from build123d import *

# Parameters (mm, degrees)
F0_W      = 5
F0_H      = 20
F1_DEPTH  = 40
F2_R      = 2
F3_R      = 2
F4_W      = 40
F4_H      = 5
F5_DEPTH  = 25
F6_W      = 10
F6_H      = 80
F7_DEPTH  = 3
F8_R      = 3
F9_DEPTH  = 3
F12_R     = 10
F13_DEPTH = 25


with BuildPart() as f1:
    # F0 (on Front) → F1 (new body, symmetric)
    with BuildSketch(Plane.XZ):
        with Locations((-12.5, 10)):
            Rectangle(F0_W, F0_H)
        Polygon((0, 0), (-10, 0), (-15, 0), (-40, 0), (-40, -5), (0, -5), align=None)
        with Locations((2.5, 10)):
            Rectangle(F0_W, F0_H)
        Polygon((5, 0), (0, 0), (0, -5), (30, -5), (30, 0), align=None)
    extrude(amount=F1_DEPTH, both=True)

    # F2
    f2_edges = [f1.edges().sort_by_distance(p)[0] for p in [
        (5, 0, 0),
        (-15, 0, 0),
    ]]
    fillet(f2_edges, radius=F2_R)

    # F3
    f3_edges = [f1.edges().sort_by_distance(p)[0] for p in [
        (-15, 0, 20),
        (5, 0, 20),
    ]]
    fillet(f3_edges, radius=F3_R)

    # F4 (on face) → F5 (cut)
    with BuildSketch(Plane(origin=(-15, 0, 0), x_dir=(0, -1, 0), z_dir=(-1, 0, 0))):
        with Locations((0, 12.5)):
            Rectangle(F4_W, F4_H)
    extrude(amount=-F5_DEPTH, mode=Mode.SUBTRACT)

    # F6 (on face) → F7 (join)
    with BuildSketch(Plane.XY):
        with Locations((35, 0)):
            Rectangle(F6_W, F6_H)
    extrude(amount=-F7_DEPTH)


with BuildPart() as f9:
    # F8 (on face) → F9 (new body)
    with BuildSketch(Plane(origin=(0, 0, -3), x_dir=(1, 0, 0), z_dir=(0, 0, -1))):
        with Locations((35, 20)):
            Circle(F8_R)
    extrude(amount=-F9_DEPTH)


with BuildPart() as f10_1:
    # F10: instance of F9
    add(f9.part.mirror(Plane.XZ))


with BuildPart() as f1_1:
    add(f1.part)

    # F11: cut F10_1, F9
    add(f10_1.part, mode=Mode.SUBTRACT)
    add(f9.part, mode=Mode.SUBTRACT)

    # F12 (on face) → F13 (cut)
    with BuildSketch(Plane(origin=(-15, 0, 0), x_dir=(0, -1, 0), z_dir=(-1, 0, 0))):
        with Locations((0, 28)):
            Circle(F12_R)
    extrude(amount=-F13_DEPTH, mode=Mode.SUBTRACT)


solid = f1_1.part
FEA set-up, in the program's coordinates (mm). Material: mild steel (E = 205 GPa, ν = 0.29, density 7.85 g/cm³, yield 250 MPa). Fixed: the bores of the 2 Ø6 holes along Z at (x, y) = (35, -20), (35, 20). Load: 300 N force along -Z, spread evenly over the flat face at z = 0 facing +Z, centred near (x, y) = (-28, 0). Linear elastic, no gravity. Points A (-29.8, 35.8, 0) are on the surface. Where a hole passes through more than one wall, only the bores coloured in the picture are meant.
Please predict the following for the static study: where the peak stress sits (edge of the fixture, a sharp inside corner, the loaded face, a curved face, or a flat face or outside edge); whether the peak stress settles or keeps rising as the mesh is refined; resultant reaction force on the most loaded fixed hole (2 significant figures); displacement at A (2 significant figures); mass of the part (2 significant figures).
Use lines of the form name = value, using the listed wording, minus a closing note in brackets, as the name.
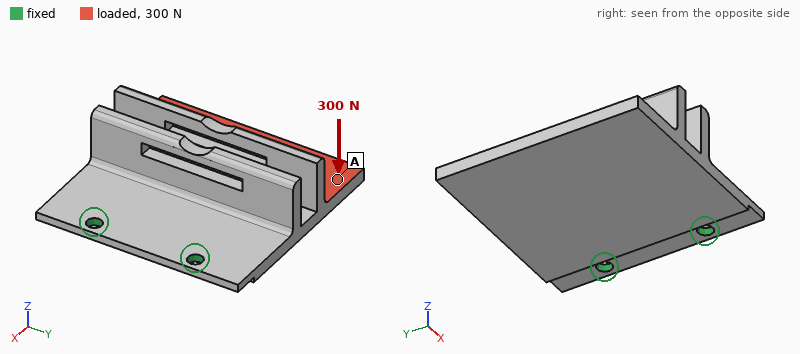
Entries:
where the peak stress sits = edge of the fixture
whether the peak stress settles or keeps rising as the mesh is refined = keeps rising
resultant reaction force on the most loaded fixed hole = 150 N
displacement at A = 0.32 mm
mass of the part = 350 g
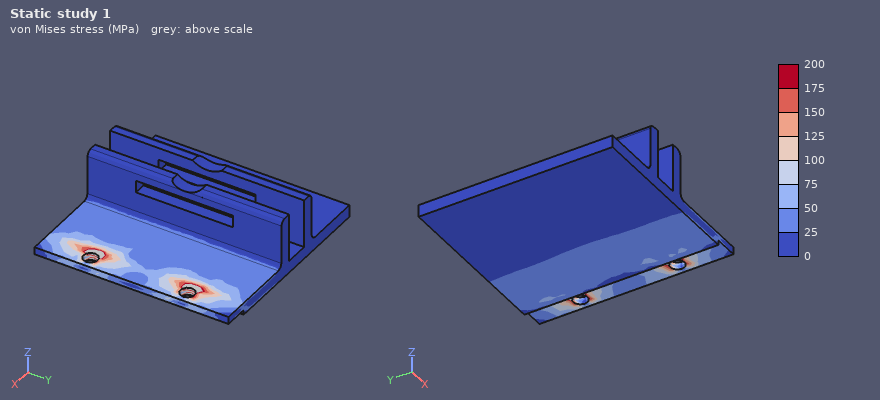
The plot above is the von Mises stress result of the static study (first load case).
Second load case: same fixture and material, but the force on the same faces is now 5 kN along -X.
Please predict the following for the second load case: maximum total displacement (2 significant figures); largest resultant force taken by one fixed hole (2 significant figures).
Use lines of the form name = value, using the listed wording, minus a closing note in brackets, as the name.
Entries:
maximum total displacement = 0.25 mm
largest resultant force taken by one fixed hole = 2.5 kN
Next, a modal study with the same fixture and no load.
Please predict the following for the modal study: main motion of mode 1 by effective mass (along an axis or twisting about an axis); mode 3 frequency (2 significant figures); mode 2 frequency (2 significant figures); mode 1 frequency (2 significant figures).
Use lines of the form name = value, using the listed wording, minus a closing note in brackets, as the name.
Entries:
main motion of mode 1 by effective mass = along Z
mode 3 frequency = 3000 Hz
mode 2 frequency = 1200 Hz
mode 1 frequency = 420 Hz
